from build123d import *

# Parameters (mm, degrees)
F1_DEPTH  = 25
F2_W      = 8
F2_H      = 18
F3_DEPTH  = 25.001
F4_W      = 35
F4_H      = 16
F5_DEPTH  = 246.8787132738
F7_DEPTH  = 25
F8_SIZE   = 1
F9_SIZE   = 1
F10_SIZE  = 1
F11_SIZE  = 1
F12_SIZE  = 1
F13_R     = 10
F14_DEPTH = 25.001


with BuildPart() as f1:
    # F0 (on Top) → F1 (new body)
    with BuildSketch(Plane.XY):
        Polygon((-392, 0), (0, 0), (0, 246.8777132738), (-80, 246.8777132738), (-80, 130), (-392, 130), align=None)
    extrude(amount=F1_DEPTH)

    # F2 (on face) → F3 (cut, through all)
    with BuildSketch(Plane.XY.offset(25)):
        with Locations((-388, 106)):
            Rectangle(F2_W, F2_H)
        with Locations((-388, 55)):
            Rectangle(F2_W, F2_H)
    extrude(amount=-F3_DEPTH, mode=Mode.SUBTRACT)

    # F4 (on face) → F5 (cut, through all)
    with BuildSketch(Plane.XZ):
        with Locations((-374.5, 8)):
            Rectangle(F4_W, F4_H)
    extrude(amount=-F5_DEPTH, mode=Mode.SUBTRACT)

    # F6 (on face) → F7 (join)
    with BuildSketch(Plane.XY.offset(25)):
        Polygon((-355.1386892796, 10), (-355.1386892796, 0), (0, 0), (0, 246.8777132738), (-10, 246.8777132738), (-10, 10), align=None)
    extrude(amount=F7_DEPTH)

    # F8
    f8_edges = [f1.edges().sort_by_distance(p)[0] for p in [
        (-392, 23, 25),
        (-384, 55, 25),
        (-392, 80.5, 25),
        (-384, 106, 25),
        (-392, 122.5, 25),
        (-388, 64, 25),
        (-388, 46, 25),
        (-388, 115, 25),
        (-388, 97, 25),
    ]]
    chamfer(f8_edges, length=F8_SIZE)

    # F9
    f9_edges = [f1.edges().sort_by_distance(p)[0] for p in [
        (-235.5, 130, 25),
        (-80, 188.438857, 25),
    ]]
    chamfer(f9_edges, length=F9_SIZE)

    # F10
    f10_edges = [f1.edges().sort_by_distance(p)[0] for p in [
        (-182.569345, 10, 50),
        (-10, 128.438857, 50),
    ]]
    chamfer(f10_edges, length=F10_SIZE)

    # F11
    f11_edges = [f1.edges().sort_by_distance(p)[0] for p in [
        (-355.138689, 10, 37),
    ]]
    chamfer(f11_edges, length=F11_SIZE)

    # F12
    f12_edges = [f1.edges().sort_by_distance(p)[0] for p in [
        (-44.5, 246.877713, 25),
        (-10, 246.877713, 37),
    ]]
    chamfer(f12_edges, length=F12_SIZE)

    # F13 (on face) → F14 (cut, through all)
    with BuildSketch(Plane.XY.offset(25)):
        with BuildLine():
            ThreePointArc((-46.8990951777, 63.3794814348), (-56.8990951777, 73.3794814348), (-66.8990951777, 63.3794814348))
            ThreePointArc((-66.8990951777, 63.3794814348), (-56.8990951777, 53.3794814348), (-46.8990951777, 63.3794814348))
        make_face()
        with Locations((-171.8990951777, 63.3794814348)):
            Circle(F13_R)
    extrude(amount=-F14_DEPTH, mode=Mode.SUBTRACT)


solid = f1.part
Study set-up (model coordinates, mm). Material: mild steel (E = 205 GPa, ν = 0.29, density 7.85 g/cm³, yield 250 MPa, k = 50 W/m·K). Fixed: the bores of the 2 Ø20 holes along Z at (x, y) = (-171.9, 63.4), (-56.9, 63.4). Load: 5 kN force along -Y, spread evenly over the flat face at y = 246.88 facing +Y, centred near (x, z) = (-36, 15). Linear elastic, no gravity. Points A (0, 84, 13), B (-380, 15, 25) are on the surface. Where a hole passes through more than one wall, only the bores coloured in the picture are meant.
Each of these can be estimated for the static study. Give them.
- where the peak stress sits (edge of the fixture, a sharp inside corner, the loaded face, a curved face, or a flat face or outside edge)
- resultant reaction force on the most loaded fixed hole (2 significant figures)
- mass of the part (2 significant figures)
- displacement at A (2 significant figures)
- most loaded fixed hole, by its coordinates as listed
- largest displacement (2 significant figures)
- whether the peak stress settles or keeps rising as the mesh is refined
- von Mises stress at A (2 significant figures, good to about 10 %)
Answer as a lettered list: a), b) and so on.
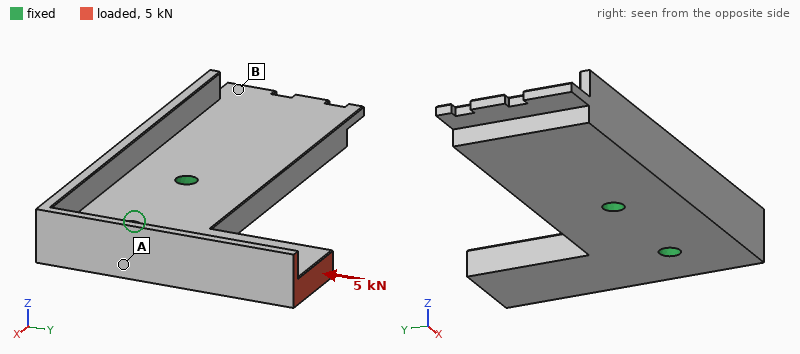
a) edge of the fixture
b) 5.6 kN
c) 12 kg
d) 1.4 µm
e) (-56.9, 63.4)
f) 4.7 µm
g) keeps rising
h) 1.6 MPa
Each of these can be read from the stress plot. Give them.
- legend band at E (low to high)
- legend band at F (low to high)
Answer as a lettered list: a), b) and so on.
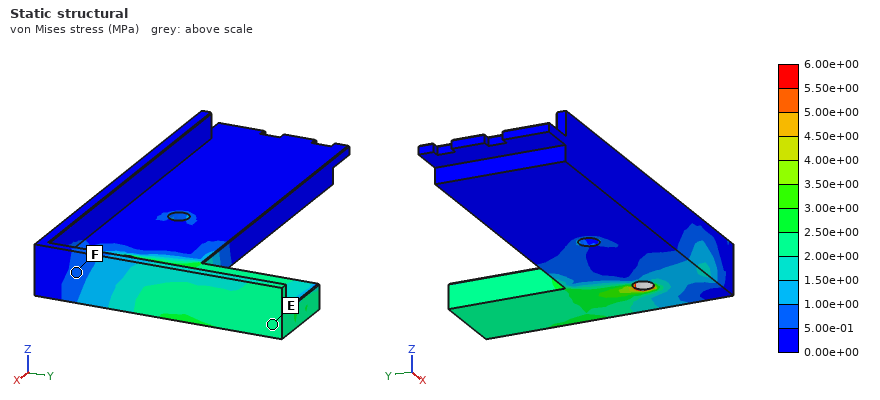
a) 2.00e+00 to 2.50e+00 MPa
b) 5.00e-01 to 1.00e+00 MPa
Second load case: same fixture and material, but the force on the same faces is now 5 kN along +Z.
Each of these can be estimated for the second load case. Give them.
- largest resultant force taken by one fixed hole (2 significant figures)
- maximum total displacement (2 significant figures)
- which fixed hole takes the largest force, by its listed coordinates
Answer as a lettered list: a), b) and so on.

a) 5.3 kN
b) 0.29 mm
c) (-56.9, 63.4)
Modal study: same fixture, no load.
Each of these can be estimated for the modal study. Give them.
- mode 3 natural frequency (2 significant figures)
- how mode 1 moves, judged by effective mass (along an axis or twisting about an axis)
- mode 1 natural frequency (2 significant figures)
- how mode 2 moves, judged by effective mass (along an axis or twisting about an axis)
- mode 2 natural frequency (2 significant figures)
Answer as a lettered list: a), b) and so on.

a) 1300 Hz
b) along Z
c) 580 Hz
d) along Z
e) 740 Hz
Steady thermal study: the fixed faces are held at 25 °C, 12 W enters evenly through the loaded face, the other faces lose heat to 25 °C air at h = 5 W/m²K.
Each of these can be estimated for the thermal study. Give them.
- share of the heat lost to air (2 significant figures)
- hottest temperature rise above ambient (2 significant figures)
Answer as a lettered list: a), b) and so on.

a) 18 %
b) 17 K
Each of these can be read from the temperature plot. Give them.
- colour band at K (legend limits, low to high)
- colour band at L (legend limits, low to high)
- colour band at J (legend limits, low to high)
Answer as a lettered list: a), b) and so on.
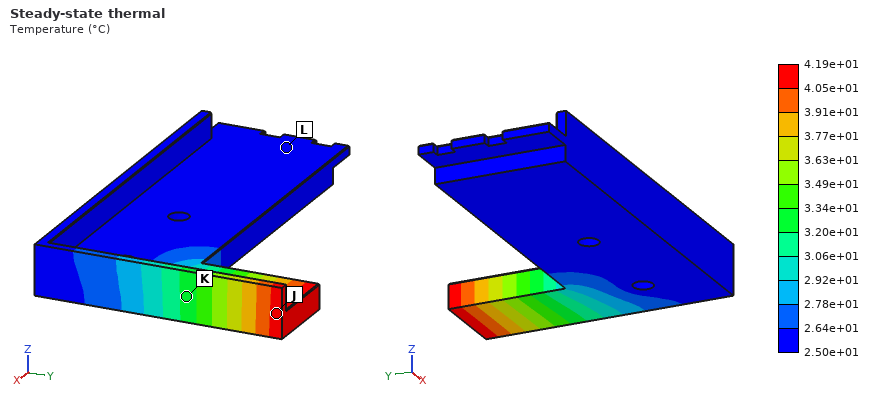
a) 3.20e+01 to 3.34e+01 °C
b) 2.50e+01 to 2.64e+01 °C
c) 4.05e+01 to 4.19e+01 °C
